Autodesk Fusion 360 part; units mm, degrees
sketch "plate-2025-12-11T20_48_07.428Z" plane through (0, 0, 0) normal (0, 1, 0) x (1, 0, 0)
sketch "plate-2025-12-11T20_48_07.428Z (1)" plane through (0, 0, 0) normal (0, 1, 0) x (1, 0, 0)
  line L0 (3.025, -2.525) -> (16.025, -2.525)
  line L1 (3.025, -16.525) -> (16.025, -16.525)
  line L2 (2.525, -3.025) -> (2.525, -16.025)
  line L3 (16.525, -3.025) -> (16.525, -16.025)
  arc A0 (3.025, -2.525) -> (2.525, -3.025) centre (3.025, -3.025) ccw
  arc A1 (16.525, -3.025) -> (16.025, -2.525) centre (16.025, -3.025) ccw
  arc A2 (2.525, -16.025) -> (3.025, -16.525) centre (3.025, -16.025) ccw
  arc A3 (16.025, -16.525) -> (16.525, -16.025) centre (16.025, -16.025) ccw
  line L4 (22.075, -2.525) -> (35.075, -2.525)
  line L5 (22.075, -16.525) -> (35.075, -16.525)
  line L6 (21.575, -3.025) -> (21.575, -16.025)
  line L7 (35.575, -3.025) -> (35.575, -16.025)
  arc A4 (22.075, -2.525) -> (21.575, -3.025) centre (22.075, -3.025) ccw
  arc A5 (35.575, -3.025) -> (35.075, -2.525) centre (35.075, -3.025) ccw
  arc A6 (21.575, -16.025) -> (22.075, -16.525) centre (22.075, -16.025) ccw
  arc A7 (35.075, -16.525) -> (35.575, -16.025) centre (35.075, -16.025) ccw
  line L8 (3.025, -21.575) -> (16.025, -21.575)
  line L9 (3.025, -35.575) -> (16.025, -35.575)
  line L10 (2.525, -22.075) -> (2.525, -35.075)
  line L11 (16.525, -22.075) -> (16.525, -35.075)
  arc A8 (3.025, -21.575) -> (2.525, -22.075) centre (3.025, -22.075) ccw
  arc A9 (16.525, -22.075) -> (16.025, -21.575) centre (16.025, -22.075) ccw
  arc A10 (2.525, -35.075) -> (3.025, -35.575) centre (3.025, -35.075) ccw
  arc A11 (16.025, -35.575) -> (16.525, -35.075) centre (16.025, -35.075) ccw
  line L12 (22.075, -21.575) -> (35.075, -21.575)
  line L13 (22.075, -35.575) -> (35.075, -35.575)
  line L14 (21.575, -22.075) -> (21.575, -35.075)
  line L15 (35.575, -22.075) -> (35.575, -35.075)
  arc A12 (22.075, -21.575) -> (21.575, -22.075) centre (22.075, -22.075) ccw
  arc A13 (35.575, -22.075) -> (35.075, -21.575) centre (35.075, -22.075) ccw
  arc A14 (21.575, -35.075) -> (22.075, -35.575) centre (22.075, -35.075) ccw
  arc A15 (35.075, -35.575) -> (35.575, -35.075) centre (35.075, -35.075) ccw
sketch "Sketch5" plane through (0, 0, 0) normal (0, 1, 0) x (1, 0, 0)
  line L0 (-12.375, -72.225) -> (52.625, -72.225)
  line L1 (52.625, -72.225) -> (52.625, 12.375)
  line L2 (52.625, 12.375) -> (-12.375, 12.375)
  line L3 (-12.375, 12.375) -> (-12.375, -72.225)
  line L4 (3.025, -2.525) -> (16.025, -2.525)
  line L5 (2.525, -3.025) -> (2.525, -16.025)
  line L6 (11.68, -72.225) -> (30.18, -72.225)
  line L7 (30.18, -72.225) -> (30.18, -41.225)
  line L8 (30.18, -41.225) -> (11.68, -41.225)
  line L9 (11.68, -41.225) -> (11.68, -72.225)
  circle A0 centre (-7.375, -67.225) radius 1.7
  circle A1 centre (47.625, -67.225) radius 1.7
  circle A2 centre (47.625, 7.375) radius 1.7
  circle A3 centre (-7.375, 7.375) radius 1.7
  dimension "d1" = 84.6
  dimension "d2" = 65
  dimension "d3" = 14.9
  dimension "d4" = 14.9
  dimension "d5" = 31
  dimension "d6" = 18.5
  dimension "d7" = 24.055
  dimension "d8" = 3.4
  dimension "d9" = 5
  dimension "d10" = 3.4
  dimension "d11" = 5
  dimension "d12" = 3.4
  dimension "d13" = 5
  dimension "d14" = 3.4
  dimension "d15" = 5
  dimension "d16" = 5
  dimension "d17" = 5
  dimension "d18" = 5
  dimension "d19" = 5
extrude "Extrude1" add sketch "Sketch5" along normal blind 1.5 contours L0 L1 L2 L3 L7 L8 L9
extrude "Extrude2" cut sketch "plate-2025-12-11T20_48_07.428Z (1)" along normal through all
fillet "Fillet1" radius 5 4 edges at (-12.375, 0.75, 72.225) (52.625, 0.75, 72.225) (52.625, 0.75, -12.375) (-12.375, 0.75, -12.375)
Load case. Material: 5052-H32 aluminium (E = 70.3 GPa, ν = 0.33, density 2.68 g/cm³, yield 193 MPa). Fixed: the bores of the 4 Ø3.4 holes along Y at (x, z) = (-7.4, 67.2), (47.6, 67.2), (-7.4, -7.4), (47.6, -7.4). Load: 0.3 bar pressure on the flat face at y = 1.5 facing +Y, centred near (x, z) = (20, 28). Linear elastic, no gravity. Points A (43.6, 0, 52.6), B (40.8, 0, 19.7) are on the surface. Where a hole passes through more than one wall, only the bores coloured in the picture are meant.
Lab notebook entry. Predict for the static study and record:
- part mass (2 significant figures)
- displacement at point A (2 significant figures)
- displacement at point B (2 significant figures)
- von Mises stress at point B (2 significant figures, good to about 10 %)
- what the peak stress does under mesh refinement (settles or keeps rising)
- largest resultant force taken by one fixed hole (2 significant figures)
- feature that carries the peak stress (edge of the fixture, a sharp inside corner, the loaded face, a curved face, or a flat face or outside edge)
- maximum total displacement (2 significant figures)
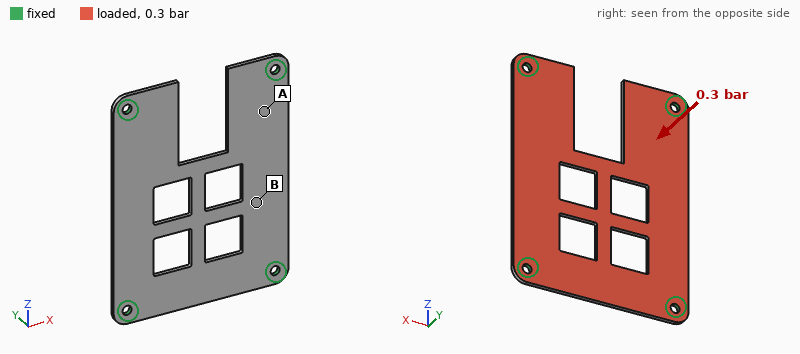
16 g
0.066 mm
0.14 mm
16 MPa
keeps rising
32 N
edge of the fixture
0.21 mm
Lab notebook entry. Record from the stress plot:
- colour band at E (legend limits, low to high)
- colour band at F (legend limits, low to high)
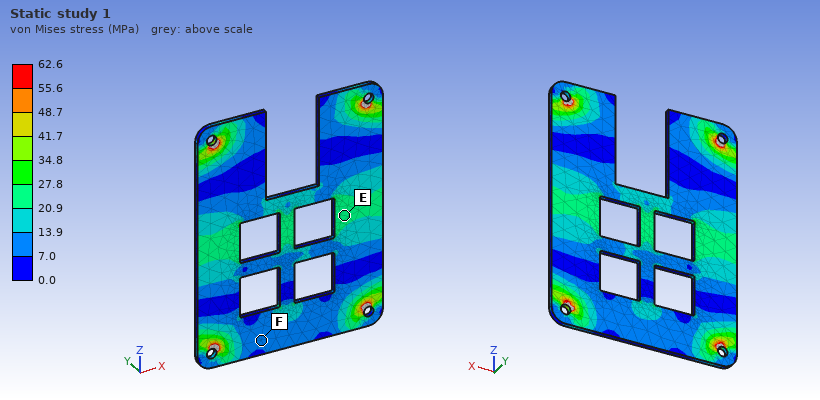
20.9 to 27.8 MPa
7.0 to 13.9 MPa
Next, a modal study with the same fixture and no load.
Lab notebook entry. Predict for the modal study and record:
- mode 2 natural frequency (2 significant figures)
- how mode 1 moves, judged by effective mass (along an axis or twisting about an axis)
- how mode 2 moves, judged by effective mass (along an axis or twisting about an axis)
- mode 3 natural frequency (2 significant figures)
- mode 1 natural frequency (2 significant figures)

1700 Hz
along Y
twisting about Z
2400 Hz
1200 Hz
